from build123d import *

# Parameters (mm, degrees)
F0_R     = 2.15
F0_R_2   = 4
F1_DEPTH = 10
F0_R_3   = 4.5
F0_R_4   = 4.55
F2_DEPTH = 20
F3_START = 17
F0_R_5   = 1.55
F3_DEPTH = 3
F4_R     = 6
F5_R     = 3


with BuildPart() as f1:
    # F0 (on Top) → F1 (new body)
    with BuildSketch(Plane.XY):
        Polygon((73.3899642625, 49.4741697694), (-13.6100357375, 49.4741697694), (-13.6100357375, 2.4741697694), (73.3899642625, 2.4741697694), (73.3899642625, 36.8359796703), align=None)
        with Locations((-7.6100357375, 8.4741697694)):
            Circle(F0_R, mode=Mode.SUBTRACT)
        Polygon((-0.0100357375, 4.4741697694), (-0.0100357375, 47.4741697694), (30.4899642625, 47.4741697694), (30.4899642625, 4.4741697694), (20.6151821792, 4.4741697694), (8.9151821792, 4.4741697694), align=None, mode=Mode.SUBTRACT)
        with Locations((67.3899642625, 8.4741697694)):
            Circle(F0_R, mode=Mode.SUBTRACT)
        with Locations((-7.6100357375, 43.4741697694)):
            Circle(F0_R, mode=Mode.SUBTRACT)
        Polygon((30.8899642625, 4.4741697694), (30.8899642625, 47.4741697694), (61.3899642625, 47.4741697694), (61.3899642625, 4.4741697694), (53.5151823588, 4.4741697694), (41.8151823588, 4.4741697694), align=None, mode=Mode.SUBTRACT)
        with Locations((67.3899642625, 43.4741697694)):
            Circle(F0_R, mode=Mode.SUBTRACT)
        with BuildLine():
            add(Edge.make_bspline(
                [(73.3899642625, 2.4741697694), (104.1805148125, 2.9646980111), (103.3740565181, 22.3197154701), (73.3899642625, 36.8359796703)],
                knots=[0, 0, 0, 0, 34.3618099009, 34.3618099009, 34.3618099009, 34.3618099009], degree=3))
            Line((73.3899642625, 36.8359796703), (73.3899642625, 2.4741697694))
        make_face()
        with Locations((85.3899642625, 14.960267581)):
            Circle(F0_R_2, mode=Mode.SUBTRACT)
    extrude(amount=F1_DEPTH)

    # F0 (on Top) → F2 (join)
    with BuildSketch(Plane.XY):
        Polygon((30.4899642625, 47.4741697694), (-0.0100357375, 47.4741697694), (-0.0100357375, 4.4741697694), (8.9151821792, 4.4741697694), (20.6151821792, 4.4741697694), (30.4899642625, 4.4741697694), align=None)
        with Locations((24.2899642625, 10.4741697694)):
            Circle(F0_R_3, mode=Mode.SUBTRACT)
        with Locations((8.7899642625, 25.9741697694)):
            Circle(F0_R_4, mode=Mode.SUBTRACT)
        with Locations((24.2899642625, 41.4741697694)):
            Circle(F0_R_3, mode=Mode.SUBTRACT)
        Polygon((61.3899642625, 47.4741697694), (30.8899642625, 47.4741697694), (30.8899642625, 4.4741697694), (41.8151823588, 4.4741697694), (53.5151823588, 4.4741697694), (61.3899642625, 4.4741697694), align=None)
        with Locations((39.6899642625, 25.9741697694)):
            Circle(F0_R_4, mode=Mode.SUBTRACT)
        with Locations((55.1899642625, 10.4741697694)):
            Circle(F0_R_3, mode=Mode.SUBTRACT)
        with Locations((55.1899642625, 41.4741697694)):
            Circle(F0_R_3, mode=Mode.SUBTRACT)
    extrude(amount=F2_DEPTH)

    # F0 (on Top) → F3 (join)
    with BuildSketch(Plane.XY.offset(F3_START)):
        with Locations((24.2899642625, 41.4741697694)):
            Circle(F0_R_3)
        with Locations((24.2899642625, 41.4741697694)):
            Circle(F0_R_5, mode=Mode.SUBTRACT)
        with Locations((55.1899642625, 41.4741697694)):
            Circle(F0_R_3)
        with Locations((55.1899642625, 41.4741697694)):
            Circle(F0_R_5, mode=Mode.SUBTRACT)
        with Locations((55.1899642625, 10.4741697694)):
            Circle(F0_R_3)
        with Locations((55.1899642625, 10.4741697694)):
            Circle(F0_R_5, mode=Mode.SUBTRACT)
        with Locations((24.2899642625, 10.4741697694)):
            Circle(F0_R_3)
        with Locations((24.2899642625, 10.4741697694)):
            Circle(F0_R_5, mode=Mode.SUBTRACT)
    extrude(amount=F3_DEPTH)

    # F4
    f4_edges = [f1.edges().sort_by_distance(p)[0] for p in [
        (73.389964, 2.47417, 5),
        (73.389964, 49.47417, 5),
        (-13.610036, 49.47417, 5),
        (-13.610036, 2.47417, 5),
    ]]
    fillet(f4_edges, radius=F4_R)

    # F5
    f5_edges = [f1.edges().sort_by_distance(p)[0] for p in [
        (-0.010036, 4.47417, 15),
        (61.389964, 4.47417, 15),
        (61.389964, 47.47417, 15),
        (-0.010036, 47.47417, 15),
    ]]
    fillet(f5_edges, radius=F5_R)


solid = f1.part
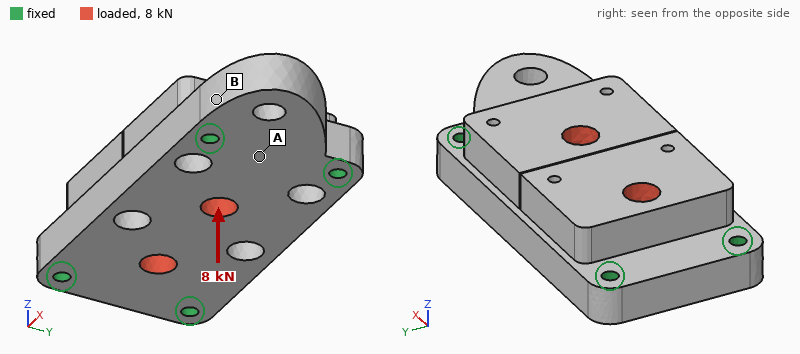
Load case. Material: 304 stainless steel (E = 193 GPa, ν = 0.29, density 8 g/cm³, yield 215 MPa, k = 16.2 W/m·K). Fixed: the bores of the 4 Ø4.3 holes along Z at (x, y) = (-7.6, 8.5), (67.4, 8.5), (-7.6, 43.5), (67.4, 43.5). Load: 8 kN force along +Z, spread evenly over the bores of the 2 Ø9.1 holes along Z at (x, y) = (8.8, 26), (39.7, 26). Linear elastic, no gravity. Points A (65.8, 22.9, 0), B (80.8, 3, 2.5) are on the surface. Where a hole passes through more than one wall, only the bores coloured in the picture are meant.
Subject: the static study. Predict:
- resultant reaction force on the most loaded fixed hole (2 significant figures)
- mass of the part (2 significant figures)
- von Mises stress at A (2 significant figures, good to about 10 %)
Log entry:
2.5 kN
510 g
19 MPa
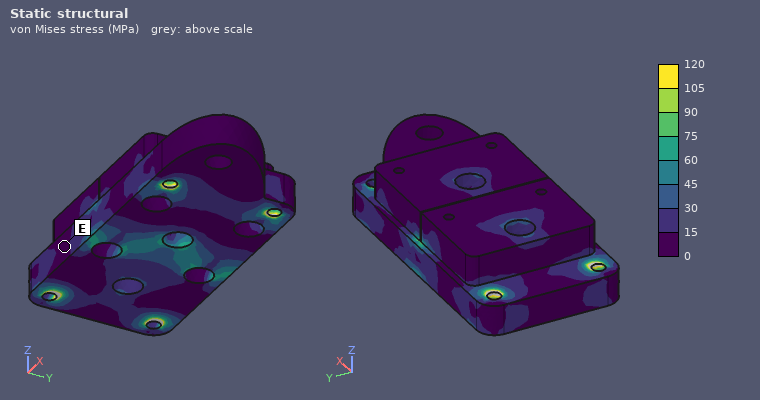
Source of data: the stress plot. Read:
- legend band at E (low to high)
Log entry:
0 to 15 MPa
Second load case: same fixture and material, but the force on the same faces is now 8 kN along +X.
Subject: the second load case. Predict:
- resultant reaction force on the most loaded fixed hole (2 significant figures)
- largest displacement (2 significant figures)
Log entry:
2.4 kN
2.9 µm
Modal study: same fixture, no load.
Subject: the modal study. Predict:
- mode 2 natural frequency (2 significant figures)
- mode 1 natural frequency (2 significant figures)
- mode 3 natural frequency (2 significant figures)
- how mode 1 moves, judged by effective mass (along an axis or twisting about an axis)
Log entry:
10 kHz
6000 Hz
11 kHz
along Z
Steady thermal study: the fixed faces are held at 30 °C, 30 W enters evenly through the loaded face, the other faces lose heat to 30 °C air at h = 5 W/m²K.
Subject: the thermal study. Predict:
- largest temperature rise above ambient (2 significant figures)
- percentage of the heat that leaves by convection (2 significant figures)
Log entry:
54 K
7.8 %
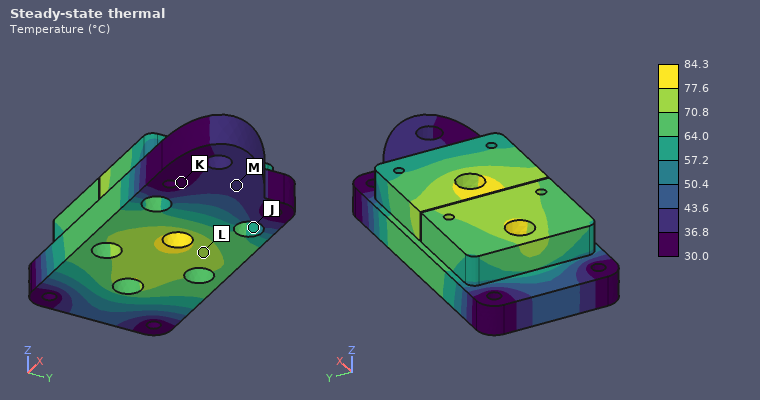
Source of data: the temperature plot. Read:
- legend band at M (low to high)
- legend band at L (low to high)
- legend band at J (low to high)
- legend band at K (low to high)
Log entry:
36.8 to 43.6 °C
70.8 to 77.6 °C
57.2 to 64.0 °C
30.0 to 36.8 °C
